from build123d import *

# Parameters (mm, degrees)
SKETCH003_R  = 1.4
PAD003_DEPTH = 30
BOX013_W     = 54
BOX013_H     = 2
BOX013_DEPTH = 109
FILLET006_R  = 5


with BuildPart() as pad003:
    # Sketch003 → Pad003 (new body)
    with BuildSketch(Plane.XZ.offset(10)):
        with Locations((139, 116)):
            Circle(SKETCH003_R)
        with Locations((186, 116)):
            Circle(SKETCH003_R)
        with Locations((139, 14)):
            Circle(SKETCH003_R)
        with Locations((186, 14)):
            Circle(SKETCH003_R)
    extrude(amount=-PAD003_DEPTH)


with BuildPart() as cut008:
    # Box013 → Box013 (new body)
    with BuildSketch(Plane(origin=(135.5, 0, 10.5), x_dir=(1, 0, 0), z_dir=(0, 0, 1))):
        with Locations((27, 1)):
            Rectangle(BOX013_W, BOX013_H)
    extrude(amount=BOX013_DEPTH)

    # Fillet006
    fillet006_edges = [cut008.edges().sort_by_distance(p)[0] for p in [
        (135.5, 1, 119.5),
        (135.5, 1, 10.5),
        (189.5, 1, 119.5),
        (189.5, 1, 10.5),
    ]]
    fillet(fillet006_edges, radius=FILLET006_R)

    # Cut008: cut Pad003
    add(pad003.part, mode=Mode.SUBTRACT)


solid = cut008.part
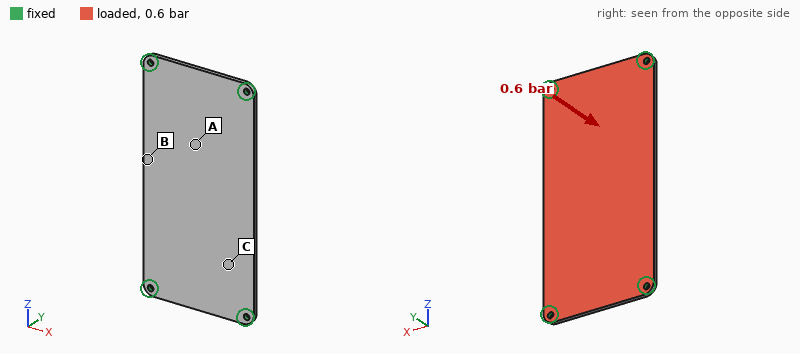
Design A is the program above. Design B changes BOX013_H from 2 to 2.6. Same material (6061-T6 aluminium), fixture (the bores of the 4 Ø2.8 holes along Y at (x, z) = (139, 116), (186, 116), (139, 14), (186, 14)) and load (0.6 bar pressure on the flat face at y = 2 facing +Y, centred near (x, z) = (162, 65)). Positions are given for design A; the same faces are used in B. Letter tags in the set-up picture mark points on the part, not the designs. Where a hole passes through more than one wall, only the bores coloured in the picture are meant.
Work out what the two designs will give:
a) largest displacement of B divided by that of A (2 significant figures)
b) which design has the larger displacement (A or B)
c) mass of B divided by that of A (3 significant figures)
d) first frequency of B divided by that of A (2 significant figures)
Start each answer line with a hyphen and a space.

- 0.47
- A
- 1.30
- 1.3
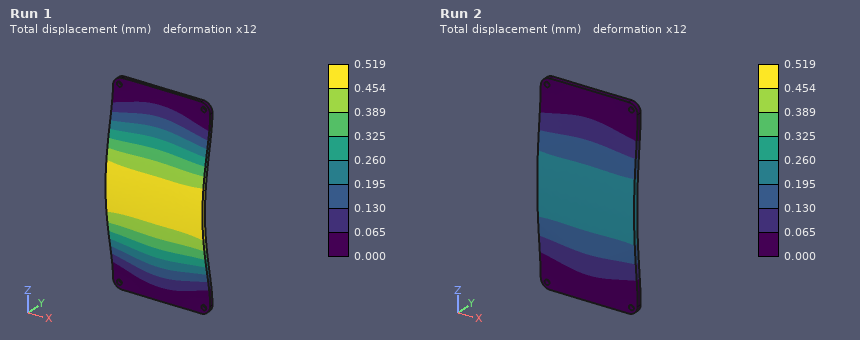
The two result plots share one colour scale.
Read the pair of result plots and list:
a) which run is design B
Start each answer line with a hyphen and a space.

- Run 2
